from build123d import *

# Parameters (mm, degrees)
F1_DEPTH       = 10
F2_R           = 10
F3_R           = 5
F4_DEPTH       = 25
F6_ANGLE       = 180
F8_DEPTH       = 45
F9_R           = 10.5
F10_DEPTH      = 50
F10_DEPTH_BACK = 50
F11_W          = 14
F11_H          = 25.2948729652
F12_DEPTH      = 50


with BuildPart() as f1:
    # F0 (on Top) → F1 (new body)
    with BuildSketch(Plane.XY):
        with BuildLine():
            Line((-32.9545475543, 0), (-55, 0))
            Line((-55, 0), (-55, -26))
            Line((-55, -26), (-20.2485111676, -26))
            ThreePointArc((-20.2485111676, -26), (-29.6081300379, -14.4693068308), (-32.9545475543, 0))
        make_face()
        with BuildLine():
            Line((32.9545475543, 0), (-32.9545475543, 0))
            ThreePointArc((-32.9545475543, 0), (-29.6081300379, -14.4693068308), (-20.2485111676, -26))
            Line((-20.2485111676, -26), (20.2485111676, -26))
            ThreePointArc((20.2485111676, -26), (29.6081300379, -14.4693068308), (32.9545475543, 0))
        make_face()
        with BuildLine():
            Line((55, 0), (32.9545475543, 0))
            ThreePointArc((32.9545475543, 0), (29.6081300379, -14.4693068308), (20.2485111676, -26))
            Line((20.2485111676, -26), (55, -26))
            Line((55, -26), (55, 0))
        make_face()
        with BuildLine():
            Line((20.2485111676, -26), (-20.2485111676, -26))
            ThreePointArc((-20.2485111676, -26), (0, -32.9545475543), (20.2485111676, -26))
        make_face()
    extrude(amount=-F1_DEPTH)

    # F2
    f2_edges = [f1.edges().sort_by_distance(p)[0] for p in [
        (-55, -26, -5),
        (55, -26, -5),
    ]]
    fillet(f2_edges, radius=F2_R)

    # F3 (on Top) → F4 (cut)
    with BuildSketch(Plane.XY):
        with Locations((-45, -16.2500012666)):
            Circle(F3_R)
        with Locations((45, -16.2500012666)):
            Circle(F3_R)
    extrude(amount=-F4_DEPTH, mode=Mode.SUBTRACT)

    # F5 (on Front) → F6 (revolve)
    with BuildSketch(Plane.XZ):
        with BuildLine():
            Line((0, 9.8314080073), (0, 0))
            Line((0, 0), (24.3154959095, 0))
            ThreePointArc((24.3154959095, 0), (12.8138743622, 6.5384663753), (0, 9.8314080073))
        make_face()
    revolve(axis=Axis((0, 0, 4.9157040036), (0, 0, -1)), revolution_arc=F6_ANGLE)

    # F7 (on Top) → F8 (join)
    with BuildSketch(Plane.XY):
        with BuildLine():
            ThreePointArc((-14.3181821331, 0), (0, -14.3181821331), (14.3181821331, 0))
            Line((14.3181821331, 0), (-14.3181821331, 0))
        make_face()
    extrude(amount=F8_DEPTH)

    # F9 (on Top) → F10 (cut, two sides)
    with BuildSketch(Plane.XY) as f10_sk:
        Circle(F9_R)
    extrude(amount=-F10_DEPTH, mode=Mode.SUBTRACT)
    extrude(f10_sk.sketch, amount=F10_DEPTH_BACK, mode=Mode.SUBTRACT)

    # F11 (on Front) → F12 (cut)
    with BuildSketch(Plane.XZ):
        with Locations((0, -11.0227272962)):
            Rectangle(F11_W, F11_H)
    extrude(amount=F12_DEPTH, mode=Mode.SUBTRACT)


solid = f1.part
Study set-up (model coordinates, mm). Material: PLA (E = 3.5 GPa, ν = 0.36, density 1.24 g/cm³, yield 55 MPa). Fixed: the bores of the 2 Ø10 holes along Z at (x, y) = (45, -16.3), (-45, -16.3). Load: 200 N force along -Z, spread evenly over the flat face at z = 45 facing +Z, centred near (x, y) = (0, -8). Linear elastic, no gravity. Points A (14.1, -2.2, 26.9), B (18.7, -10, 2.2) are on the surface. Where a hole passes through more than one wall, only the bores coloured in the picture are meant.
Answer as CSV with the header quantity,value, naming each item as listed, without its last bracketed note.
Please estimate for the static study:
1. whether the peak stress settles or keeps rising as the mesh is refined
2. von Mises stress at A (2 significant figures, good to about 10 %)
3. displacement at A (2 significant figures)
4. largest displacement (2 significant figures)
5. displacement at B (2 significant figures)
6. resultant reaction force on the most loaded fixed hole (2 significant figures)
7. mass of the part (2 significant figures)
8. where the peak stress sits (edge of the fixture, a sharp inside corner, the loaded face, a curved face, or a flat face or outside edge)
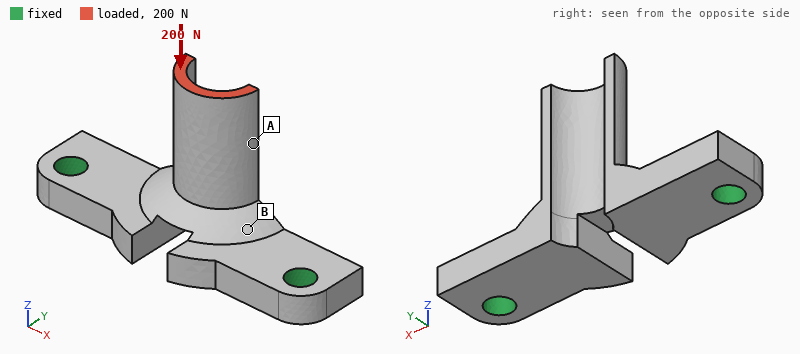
quantity,value
whether the peak stress settles or keeps rising as the mesh is refined,keeps rising
von Mises stress at A,1.2 MPa
displacement at A,0.10 mm
largest displacement,0.12 mm
displacement at B,0.058 mm
resultant reaction force on the most loaded fixed hole,170 N
mass of the part,39 g
where the peak stress sits,edge of the fixture
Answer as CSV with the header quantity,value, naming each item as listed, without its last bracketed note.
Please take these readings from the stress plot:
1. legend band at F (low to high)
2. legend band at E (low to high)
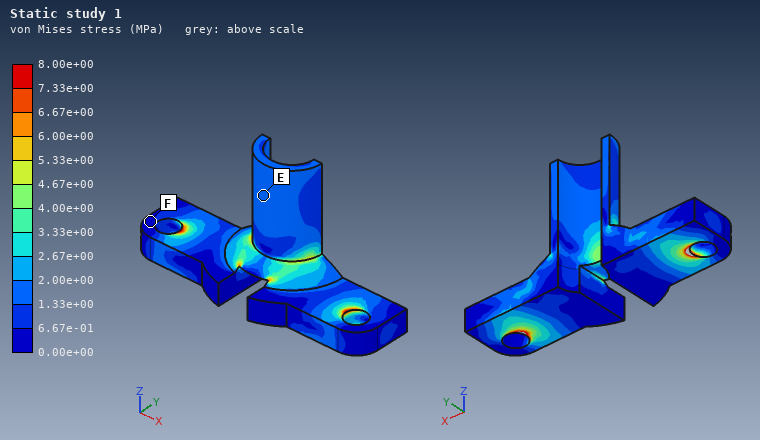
quantity,value
legend band at F,0.00e+00 to 6.67e-01 MPa
legend band at E,1.33e+00 to 2.00e+00 MPa
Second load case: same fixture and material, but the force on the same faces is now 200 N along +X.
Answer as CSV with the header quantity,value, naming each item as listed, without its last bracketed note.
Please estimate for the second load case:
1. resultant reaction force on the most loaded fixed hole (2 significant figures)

quantity,value
resultant reaction force on the most loaded fixed hole,220 N
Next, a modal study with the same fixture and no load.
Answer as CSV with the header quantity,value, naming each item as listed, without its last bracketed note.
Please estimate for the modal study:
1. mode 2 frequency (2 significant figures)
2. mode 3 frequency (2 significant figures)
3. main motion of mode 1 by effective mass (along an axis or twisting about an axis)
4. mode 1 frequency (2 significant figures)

quantity,value
mode 2 frequency,1300 Hz
mode 3 frequency,1800 Hz
main motion of mode 1 by effective mass,along Y
mode 1 frequency,1000 Hz
